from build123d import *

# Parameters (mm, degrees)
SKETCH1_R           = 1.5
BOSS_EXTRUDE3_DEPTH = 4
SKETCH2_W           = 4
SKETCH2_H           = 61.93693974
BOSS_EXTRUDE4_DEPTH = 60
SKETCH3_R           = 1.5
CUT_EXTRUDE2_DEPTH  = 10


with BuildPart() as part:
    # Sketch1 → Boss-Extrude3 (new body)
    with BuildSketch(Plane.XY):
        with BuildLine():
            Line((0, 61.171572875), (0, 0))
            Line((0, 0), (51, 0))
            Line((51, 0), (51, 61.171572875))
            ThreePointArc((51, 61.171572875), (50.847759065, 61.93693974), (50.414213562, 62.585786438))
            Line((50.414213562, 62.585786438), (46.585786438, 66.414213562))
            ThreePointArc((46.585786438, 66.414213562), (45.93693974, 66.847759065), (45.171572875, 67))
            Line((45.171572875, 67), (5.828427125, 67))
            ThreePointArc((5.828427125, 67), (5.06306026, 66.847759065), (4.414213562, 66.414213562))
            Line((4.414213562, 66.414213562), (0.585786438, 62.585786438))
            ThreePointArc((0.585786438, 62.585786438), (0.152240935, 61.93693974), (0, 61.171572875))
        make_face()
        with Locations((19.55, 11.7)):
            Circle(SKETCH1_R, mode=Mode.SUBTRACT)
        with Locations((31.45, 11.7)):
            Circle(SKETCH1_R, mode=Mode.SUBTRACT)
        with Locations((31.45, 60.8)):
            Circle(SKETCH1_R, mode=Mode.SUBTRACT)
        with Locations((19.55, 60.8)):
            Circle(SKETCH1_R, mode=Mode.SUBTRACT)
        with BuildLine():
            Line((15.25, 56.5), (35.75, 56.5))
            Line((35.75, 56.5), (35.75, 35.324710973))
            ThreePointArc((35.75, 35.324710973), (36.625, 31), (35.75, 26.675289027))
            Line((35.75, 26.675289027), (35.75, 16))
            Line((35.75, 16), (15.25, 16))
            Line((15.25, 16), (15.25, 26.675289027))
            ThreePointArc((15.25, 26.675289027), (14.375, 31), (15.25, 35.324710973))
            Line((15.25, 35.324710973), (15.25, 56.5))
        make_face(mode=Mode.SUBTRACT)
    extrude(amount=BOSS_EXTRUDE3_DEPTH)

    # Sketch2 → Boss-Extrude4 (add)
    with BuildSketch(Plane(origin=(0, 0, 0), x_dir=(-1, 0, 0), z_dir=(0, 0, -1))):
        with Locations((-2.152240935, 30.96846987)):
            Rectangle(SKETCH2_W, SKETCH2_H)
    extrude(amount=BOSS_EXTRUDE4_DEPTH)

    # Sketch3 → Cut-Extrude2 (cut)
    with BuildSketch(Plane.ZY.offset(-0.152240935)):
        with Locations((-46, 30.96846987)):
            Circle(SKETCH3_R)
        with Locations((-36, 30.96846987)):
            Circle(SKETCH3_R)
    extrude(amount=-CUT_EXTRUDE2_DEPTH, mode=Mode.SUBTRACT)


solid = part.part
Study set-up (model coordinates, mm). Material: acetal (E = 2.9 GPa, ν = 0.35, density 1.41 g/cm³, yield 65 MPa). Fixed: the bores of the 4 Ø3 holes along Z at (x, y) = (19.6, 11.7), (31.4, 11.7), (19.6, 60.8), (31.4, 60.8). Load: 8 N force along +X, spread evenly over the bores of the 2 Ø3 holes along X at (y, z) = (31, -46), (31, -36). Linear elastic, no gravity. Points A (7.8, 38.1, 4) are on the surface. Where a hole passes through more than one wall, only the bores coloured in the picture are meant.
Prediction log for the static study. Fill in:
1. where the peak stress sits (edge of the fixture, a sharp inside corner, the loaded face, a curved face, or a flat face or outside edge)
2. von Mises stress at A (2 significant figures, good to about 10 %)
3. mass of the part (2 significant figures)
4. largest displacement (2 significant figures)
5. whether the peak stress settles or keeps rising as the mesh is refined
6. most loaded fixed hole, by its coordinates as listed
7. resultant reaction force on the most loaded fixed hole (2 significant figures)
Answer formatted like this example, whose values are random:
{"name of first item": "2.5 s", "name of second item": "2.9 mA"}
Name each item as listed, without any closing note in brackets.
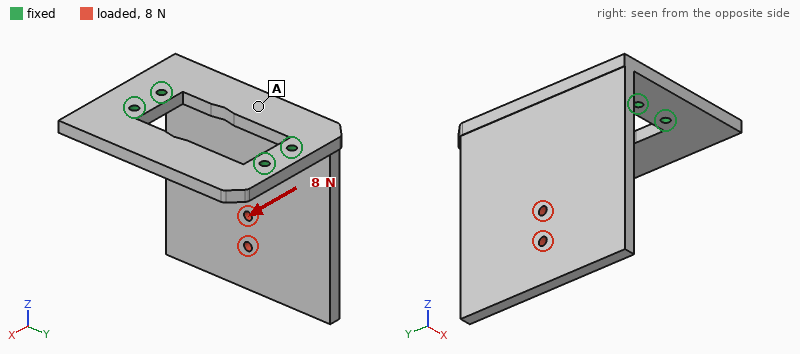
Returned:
{"where the peak stress sits": "edge of the fixture", "von Mises stress at A": "0.77 MPa", "mass of the part": "35 g", "largest displacement": "1.1 mm", "whether the peak stress settles or keeps rising as the mesh is refined": "keeps rising", "most loaded fixed hole, by its coordinates as listed": "(19.6, 11.7)", "resultant reaction force on the most loaded fixed hole": "7.9 N"}
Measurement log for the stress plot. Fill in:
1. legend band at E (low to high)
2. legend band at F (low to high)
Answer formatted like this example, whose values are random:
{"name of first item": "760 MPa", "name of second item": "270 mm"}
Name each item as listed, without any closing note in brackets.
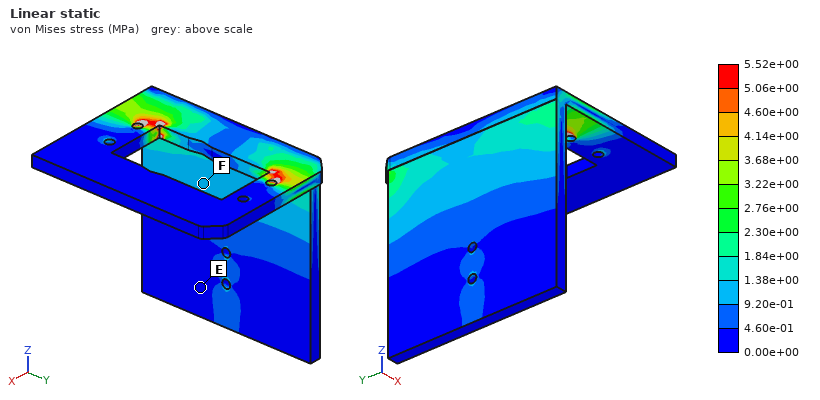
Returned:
{"legend band at E": "0.00e+00 to 4.60e-01 MPa", "legend band at F": "9.20e-01 to 1.38e+00 MPa"}
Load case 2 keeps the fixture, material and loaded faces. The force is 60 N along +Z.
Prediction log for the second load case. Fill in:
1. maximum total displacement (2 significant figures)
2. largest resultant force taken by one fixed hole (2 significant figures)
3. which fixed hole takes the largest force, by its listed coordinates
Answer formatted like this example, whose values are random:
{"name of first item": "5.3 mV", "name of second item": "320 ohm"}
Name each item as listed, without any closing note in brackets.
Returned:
{"maximum total displacement": "1.2 mm", "largest resultant force taken by one fixed hole": "51 N", "which fixed hole takes the largest force, by its listed coordinates": "(19.6, 11.7)"}
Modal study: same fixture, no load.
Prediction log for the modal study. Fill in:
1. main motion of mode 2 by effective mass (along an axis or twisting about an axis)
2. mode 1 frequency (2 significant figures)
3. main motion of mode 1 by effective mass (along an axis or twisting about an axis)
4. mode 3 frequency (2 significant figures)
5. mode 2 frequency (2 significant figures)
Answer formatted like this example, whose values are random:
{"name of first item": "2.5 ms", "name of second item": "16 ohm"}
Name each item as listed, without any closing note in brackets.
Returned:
{"main motion of mode 2 by effective mass": "along Y", "mode 1 frequency": "140 Hz", "main motion of mode 1 by effective mass": "along X", "mode 3 frequency": "620 Hz", "mode 2 frequency": "430 Hz"}
